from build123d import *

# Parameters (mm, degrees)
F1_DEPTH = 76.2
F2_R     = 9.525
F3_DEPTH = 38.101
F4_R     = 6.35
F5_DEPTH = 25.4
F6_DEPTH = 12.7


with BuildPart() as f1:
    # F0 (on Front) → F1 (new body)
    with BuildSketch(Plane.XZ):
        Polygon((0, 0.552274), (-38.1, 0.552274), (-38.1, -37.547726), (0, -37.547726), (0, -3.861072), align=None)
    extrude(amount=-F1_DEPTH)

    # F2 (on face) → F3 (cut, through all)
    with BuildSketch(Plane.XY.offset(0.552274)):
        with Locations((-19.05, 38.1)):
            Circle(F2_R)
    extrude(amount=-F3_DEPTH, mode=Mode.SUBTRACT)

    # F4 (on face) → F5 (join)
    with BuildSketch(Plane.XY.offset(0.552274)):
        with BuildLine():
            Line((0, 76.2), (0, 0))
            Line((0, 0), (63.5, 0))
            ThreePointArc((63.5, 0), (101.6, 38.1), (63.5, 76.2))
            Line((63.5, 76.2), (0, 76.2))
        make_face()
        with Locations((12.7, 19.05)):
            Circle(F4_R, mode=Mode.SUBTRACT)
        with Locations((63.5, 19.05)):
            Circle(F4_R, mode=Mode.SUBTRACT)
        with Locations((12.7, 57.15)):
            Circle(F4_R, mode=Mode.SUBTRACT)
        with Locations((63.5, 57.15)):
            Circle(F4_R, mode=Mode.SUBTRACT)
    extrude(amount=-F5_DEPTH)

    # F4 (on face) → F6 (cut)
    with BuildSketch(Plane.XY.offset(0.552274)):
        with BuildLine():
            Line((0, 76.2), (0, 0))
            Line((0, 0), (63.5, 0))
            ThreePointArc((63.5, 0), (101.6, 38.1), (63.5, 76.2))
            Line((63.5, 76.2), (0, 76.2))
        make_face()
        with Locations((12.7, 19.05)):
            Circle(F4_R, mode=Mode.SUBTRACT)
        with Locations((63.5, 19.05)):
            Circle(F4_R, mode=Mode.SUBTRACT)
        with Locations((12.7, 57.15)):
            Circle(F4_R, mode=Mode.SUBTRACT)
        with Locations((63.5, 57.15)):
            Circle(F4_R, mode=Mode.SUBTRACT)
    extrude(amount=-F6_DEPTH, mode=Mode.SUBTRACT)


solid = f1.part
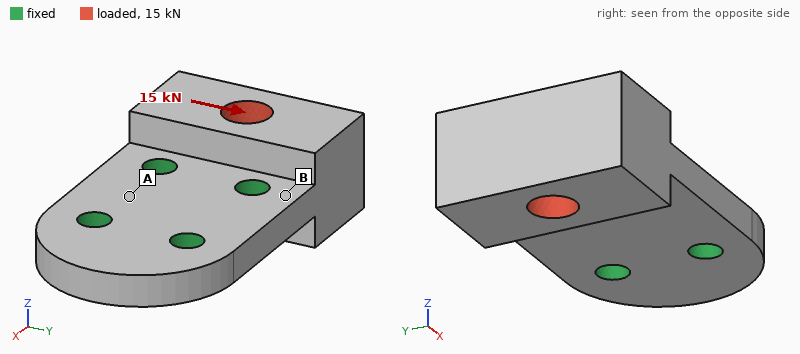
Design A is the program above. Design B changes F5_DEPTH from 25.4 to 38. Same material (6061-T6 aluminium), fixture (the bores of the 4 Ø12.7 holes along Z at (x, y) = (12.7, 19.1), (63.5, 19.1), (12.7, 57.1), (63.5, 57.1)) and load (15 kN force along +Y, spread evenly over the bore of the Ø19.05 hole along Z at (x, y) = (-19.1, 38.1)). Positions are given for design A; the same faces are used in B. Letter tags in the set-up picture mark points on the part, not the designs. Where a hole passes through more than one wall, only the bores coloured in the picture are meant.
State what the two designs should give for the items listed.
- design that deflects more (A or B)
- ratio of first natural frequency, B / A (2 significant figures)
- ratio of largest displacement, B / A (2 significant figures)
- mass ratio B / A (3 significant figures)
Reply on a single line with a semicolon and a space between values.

A; 2.2; 0.70; 1.45
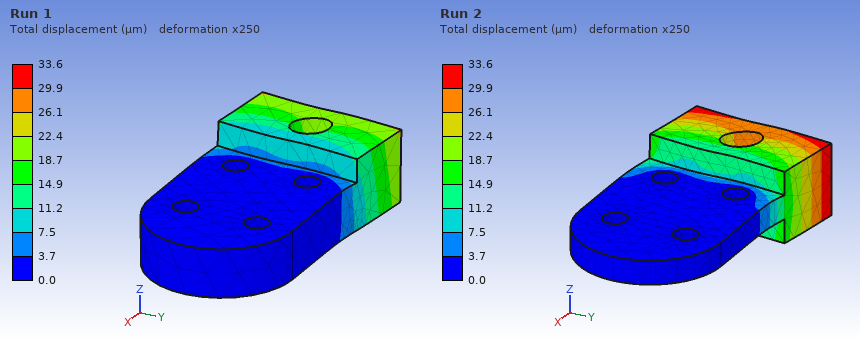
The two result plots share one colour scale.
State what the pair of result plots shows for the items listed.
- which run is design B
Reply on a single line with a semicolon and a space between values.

Run 1
